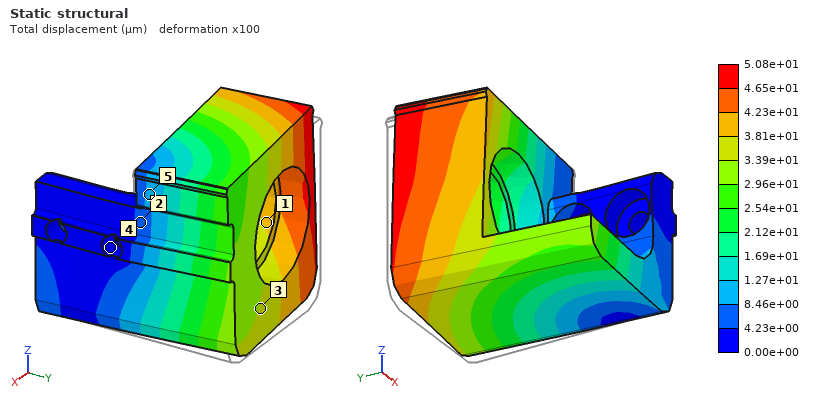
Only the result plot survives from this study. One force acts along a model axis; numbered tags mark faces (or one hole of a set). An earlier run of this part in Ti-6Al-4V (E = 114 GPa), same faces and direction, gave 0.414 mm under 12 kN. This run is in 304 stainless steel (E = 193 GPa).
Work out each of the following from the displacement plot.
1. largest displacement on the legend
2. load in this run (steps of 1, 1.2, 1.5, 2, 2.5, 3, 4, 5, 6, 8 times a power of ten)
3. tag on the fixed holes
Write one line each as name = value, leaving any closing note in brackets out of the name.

largest displacement on the legend = 5.08e+01 µm
load in this run = 2.5 kN
tag on the fixed holes = 4
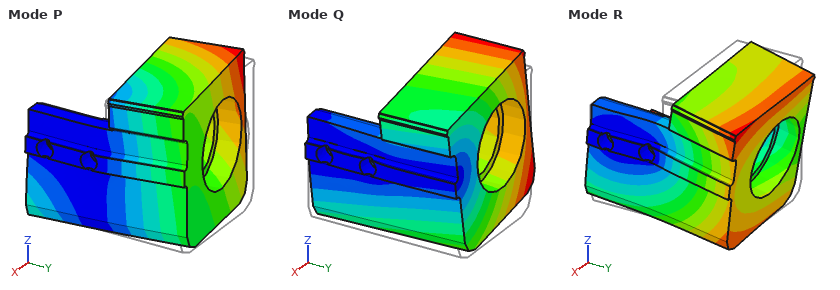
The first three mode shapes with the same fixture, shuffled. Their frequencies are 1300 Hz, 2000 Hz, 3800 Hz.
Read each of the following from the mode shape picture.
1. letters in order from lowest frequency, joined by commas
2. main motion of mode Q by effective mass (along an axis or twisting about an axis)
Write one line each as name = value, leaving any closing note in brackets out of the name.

letters in order from lowest frequency, joined by commas = Q, P, R
main motion of mode Q by effective mass = along Z
